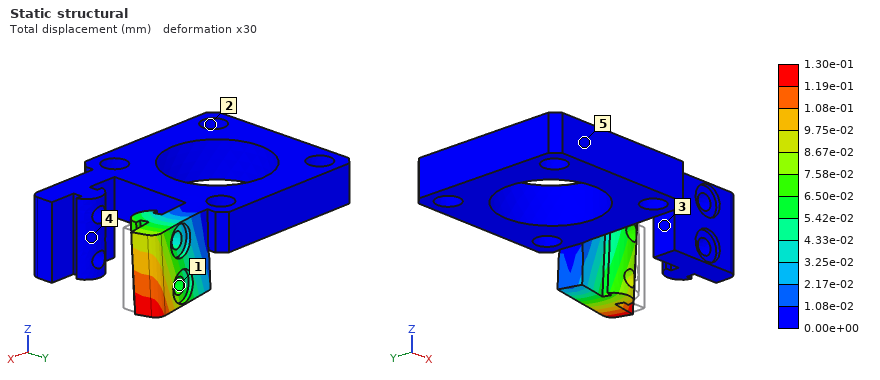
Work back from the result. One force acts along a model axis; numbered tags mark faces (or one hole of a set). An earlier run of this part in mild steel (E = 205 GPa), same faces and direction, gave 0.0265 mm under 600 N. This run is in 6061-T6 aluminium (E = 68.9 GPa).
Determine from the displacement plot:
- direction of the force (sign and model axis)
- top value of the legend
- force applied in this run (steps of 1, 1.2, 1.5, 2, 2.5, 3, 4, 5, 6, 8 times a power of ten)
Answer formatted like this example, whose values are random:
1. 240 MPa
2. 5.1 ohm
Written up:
1. +Y
2. 1.30e-01 mm
3. 1 kN
